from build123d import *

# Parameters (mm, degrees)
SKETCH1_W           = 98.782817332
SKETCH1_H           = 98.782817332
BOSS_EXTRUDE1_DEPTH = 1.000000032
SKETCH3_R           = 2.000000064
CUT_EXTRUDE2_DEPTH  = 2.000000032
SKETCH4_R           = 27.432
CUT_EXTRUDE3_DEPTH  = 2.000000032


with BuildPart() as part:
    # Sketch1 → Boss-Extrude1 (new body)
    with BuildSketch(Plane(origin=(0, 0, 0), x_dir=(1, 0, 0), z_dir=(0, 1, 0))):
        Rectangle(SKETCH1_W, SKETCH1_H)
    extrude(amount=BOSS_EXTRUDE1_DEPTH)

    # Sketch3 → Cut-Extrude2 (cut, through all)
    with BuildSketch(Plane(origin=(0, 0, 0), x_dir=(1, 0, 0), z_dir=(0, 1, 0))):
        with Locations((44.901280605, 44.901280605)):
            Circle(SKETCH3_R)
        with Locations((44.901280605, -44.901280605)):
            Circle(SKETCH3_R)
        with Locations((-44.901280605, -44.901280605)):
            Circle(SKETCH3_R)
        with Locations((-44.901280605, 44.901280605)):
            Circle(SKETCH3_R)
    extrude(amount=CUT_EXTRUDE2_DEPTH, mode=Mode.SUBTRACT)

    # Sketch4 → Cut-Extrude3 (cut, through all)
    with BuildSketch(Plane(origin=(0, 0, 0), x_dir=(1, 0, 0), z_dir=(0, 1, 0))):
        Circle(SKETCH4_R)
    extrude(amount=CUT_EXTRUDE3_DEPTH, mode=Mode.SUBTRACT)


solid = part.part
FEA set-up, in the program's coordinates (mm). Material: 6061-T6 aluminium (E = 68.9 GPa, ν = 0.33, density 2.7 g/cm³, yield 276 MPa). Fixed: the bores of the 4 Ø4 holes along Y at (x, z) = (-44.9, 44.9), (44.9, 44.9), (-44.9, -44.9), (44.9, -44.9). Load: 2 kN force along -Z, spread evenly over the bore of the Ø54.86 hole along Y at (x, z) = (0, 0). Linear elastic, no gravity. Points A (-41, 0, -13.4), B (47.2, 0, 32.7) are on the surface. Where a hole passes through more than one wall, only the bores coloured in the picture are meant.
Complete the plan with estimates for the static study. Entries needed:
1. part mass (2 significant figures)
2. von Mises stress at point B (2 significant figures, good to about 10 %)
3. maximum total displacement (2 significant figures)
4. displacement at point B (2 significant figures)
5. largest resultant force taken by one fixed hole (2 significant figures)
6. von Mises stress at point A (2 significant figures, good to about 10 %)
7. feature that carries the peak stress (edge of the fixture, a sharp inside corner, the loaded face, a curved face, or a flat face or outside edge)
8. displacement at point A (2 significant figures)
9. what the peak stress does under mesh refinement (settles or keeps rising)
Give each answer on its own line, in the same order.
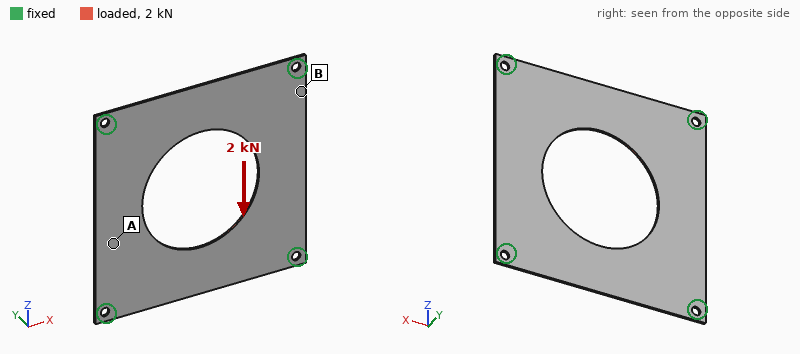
20 g
31 MPa
32 µm
5.9 µm
550 N
18 MPa
edge of the fixture
14 µm
keeps rising
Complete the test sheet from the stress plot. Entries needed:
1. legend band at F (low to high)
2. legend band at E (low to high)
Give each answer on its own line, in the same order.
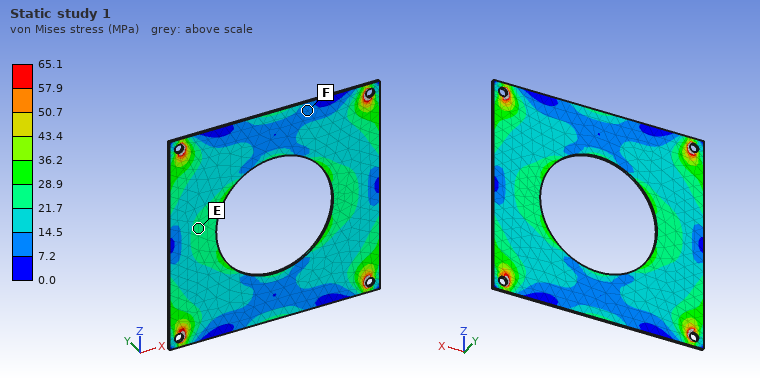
7.2 to 14.5 MPa
21.7 to 28.9 MPa
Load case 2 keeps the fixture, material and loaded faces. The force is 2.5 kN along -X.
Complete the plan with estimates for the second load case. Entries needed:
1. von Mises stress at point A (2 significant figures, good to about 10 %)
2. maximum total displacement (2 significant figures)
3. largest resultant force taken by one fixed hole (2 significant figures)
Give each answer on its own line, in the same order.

16 MPa
40 µm
690 N
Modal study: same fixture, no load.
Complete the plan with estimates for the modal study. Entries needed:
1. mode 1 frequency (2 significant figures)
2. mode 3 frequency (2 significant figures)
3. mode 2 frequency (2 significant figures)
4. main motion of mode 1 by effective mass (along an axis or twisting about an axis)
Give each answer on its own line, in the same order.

490 Hz
690 Hz
690 Hz
along Y
